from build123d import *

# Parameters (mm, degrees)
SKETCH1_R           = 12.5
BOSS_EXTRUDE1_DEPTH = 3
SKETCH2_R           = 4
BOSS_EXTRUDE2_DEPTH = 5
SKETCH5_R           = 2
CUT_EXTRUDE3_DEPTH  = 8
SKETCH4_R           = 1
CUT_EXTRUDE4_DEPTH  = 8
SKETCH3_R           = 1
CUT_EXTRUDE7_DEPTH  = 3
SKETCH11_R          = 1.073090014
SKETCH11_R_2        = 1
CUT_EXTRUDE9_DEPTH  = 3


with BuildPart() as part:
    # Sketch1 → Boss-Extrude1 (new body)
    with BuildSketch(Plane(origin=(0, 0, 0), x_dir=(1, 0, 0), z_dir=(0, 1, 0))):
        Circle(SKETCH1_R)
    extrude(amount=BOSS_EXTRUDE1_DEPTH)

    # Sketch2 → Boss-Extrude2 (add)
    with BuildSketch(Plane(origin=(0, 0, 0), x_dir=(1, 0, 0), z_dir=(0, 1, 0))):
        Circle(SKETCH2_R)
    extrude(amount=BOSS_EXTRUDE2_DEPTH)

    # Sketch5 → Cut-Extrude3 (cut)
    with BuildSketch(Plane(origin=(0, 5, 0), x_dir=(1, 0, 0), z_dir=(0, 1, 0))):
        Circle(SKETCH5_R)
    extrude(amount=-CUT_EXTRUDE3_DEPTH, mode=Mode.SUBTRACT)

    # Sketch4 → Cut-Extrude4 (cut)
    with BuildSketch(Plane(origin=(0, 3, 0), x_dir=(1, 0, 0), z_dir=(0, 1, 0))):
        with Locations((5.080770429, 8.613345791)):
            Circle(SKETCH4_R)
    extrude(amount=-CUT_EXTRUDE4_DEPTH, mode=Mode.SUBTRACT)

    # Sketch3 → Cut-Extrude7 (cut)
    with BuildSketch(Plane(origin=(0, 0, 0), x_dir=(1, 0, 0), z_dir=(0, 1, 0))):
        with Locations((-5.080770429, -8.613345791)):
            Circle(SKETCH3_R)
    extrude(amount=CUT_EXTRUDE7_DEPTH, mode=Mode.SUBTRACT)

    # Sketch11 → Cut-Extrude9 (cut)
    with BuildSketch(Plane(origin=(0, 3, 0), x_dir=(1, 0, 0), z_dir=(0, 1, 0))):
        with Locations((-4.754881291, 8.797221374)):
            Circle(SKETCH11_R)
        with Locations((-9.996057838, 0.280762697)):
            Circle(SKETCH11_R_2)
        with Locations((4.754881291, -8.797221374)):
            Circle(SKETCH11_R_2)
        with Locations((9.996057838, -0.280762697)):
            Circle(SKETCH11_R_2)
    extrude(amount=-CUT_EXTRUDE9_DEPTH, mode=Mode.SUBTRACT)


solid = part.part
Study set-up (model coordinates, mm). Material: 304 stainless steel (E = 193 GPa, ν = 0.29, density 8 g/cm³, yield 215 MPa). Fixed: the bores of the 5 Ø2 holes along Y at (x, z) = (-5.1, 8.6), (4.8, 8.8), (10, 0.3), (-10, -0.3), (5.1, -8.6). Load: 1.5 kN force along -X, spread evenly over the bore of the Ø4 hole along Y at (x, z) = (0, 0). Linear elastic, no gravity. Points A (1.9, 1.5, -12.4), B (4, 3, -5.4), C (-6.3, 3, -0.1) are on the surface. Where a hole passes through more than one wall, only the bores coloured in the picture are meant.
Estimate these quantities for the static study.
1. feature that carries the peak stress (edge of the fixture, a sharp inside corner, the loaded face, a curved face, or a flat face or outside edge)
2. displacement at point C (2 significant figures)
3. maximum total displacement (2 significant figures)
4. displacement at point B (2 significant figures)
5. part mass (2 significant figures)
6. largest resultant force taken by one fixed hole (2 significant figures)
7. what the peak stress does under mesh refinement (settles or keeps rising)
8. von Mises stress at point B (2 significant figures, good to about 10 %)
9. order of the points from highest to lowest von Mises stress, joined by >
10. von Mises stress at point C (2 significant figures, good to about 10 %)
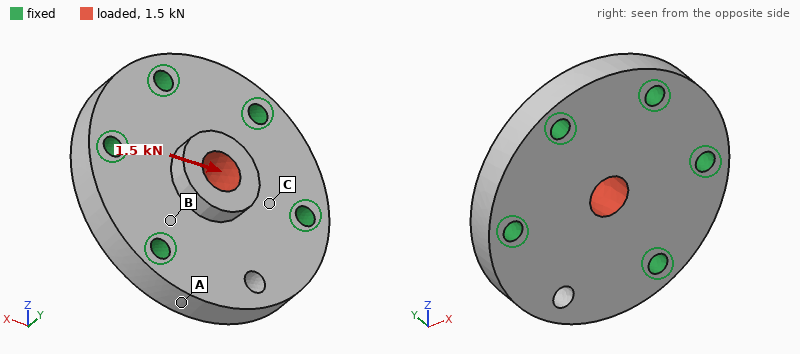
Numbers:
edge of the fixture
0.50 µm
2.1 µm
0.45 µm
12 g
430 N
keeps rising
17 MPa
C > B > A
37 MPa
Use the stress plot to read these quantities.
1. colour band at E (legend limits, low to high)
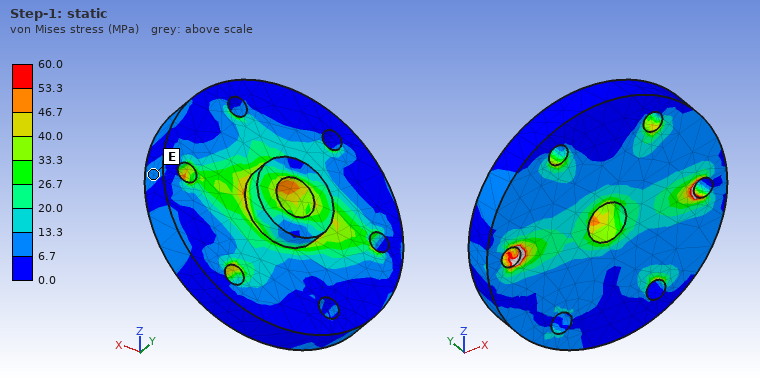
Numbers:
6.7 to 13.3 MPa
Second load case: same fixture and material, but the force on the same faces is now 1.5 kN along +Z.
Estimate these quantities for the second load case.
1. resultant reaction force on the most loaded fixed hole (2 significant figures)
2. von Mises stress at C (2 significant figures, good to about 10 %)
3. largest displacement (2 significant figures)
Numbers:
410 N
16 MPa
2.3 µm
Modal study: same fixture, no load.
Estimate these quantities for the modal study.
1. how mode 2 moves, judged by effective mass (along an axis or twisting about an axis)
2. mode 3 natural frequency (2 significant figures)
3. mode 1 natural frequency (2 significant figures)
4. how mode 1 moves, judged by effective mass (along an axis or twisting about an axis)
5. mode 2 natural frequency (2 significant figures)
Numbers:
along Y
73 kHz
33 kHz
along Y
52 kHz
